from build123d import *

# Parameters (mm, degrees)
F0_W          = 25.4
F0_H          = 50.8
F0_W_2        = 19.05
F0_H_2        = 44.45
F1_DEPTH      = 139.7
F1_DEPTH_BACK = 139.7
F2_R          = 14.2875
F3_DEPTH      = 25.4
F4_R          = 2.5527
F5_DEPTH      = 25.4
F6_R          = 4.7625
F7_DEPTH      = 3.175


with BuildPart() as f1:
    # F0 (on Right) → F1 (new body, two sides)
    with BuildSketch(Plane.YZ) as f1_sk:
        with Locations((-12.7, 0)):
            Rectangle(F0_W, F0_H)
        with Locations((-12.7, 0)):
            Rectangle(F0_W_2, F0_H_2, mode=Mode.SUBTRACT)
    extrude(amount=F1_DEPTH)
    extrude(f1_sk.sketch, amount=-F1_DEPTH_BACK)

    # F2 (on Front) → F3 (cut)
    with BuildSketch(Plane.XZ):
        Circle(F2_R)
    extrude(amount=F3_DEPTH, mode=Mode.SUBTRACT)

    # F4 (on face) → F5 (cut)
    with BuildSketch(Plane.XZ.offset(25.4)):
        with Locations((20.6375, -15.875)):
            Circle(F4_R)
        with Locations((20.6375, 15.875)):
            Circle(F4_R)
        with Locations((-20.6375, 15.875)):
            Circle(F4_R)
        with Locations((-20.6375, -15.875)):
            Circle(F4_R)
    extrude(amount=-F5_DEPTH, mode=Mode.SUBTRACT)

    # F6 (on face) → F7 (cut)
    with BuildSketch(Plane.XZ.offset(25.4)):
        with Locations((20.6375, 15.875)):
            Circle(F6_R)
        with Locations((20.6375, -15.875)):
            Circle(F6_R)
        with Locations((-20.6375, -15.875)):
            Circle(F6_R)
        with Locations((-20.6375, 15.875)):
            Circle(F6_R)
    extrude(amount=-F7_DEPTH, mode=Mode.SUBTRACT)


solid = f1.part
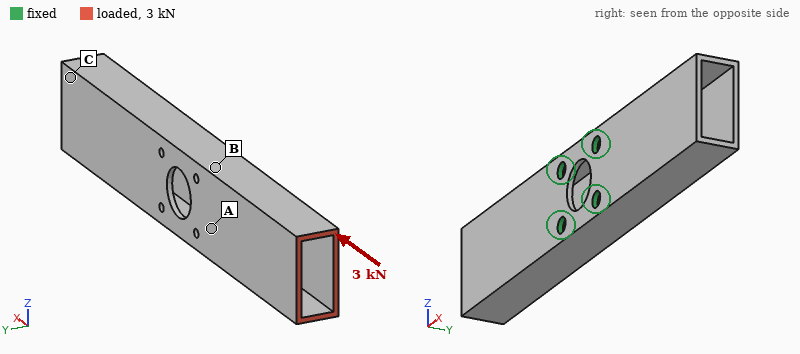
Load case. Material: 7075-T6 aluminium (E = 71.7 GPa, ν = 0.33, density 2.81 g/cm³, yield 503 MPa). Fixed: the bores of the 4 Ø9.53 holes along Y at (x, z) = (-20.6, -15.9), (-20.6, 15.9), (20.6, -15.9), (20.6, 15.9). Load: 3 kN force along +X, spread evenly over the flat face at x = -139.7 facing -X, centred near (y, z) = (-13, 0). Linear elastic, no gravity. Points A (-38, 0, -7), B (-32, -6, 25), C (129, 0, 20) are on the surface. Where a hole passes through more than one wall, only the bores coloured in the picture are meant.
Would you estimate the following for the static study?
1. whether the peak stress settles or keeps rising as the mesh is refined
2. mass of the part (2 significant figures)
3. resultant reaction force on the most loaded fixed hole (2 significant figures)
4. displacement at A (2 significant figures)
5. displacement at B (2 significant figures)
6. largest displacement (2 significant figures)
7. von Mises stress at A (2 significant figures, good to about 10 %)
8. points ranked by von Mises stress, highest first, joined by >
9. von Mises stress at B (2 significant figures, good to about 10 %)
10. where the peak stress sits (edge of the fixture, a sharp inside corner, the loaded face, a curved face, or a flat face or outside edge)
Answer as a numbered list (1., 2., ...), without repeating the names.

1. keeps rising
2. 330 g
3. 1.1 kN
4. 18 µm
5. 12 µm
6. 64 µm
7. 5.5 MPa
8. B > A > C
9. 9.3 MPa
10. edge of the fixture
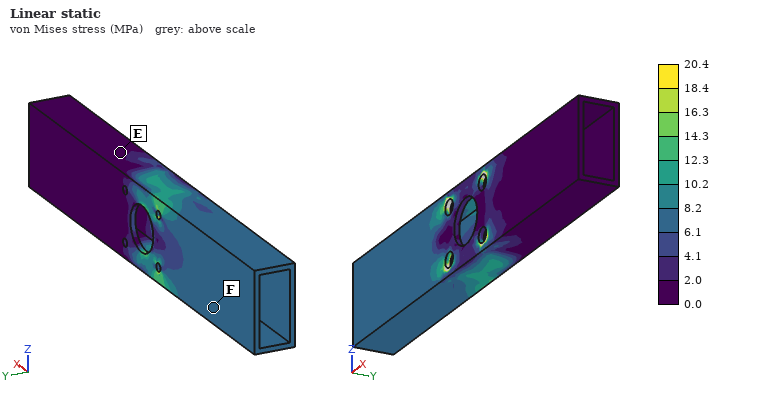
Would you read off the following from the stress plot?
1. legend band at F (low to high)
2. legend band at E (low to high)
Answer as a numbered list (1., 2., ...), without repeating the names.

1. 6.1 to 8.2 MPa
2. 0.0 to 2.0 MPa
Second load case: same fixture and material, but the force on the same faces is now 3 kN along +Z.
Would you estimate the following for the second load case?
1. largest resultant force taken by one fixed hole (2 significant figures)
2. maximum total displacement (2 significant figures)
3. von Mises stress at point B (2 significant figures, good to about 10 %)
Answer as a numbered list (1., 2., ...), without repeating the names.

1. 7.2 kN
2. 0.37 mm
3. 47 MPa
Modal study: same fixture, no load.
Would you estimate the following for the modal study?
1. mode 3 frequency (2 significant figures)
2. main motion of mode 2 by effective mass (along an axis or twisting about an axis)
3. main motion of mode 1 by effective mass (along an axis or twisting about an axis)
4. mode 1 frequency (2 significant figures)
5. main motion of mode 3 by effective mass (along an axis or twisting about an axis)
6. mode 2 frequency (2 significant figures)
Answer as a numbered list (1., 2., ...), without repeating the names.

1. 1700 Hz
2. along Y
3. twisting about Z
4. 960 Hz
5. along Z
6. 1400 Hz
